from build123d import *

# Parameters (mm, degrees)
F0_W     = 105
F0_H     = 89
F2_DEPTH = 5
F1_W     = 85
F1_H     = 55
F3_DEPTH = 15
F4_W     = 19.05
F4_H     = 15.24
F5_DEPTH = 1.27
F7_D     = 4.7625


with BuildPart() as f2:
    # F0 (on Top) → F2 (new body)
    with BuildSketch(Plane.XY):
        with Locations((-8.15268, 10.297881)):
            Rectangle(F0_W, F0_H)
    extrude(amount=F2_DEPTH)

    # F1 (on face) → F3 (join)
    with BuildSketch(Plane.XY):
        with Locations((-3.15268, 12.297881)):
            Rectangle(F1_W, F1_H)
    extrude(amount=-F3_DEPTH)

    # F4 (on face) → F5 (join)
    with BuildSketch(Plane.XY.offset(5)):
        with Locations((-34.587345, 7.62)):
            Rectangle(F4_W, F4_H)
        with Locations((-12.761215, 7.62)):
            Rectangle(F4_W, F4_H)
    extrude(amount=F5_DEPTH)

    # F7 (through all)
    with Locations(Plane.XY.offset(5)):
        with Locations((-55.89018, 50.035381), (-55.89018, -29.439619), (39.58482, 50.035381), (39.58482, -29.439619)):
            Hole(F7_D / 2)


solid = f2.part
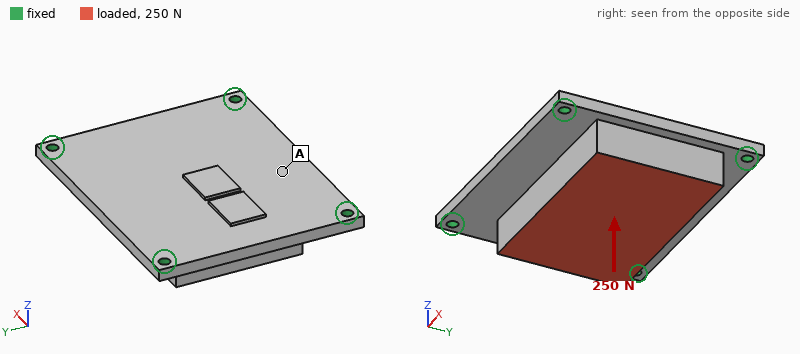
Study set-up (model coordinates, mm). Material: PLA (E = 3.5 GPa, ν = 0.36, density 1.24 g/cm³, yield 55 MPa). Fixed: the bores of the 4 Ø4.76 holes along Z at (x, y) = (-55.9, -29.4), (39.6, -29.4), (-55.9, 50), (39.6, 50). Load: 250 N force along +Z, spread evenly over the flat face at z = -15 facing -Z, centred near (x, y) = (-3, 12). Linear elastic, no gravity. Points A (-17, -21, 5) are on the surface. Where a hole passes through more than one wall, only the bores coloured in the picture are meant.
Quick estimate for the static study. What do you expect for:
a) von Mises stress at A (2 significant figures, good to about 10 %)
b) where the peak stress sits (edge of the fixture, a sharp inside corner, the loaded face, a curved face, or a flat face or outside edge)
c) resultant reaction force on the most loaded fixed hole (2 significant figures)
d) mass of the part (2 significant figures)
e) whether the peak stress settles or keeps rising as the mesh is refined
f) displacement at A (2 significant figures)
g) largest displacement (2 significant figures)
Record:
0.70 MPa
edge of the fixture
88 N
150 g
keeps rising
71 µm
72 µm
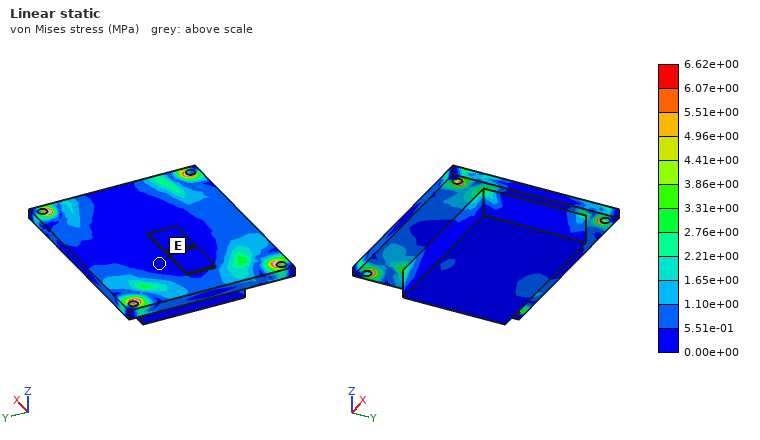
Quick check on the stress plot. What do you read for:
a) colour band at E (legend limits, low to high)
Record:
0.00e+00 to 5.51e-01 MPa
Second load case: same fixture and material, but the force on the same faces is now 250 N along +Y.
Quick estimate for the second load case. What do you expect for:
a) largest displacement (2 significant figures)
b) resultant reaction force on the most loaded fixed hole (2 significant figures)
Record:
39 µm
90 N
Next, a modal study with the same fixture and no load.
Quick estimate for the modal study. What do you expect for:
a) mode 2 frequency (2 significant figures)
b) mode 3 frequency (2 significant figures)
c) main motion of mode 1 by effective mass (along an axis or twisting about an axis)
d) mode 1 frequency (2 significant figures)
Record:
1500 Hz
1600 Hz
along Z
870 Hz
